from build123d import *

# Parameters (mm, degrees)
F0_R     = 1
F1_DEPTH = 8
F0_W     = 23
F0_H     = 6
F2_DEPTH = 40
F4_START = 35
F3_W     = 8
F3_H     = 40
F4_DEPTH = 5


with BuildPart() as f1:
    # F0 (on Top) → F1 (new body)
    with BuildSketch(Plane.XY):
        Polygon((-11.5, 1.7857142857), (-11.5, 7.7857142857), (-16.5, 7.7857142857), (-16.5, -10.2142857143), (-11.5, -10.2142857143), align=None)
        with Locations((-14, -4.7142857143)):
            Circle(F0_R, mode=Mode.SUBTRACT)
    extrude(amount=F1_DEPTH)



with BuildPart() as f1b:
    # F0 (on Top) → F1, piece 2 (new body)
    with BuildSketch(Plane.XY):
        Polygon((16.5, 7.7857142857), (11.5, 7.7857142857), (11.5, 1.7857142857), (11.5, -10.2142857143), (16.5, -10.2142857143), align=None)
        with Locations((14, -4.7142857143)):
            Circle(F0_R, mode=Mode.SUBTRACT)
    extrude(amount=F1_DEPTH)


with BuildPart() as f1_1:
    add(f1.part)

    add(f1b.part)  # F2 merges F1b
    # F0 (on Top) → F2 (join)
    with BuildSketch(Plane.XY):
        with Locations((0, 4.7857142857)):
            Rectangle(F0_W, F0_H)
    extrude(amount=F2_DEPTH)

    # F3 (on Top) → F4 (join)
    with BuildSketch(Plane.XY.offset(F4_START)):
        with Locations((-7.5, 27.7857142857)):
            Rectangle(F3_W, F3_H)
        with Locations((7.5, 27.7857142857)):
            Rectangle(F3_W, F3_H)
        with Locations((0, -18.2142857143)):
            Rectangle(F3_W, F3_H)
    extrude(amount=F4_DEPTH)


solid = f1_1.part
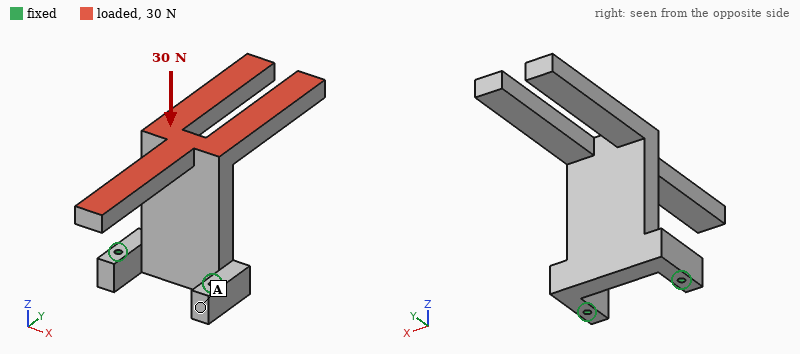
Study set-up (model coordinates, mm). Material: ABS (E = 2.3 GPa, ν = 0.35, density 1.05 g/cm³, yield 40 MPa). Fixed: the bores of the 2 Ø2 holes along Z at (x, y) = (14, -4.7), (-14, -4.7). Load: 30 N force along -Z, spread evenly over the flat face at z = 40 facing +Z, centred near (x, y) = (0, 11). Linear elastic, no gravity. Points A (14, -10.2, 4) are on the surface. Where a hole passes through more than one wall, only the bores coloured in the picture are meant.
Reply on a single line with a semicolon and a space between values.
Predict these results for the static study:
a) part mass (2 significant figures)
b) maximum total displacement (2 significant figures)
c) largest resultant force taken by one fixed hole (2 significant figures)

12 g; 0.99 mm; 15 N
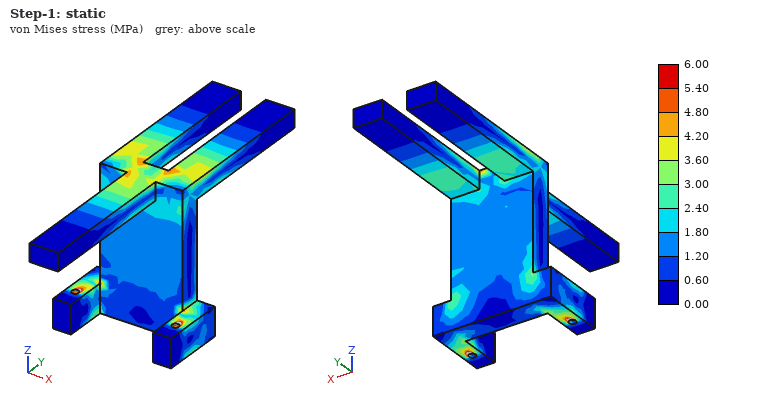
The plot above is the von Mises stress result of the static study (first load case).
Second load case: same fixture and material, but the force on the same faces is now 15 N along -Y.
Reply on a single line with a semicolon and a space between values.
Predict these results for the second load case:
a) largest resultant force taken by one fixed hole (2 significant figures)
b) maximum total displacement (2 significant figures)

9.8 N; 0.94 mm
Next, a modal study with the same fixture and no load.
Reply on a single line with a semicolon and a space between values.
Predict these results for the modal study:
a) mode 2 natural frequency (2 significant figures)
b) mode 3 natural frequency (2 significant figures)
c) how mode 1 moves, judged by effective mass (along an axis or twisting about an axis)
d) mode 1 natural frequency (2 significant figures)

490 Hz; 640 Hz; along Y; 270 Hz
